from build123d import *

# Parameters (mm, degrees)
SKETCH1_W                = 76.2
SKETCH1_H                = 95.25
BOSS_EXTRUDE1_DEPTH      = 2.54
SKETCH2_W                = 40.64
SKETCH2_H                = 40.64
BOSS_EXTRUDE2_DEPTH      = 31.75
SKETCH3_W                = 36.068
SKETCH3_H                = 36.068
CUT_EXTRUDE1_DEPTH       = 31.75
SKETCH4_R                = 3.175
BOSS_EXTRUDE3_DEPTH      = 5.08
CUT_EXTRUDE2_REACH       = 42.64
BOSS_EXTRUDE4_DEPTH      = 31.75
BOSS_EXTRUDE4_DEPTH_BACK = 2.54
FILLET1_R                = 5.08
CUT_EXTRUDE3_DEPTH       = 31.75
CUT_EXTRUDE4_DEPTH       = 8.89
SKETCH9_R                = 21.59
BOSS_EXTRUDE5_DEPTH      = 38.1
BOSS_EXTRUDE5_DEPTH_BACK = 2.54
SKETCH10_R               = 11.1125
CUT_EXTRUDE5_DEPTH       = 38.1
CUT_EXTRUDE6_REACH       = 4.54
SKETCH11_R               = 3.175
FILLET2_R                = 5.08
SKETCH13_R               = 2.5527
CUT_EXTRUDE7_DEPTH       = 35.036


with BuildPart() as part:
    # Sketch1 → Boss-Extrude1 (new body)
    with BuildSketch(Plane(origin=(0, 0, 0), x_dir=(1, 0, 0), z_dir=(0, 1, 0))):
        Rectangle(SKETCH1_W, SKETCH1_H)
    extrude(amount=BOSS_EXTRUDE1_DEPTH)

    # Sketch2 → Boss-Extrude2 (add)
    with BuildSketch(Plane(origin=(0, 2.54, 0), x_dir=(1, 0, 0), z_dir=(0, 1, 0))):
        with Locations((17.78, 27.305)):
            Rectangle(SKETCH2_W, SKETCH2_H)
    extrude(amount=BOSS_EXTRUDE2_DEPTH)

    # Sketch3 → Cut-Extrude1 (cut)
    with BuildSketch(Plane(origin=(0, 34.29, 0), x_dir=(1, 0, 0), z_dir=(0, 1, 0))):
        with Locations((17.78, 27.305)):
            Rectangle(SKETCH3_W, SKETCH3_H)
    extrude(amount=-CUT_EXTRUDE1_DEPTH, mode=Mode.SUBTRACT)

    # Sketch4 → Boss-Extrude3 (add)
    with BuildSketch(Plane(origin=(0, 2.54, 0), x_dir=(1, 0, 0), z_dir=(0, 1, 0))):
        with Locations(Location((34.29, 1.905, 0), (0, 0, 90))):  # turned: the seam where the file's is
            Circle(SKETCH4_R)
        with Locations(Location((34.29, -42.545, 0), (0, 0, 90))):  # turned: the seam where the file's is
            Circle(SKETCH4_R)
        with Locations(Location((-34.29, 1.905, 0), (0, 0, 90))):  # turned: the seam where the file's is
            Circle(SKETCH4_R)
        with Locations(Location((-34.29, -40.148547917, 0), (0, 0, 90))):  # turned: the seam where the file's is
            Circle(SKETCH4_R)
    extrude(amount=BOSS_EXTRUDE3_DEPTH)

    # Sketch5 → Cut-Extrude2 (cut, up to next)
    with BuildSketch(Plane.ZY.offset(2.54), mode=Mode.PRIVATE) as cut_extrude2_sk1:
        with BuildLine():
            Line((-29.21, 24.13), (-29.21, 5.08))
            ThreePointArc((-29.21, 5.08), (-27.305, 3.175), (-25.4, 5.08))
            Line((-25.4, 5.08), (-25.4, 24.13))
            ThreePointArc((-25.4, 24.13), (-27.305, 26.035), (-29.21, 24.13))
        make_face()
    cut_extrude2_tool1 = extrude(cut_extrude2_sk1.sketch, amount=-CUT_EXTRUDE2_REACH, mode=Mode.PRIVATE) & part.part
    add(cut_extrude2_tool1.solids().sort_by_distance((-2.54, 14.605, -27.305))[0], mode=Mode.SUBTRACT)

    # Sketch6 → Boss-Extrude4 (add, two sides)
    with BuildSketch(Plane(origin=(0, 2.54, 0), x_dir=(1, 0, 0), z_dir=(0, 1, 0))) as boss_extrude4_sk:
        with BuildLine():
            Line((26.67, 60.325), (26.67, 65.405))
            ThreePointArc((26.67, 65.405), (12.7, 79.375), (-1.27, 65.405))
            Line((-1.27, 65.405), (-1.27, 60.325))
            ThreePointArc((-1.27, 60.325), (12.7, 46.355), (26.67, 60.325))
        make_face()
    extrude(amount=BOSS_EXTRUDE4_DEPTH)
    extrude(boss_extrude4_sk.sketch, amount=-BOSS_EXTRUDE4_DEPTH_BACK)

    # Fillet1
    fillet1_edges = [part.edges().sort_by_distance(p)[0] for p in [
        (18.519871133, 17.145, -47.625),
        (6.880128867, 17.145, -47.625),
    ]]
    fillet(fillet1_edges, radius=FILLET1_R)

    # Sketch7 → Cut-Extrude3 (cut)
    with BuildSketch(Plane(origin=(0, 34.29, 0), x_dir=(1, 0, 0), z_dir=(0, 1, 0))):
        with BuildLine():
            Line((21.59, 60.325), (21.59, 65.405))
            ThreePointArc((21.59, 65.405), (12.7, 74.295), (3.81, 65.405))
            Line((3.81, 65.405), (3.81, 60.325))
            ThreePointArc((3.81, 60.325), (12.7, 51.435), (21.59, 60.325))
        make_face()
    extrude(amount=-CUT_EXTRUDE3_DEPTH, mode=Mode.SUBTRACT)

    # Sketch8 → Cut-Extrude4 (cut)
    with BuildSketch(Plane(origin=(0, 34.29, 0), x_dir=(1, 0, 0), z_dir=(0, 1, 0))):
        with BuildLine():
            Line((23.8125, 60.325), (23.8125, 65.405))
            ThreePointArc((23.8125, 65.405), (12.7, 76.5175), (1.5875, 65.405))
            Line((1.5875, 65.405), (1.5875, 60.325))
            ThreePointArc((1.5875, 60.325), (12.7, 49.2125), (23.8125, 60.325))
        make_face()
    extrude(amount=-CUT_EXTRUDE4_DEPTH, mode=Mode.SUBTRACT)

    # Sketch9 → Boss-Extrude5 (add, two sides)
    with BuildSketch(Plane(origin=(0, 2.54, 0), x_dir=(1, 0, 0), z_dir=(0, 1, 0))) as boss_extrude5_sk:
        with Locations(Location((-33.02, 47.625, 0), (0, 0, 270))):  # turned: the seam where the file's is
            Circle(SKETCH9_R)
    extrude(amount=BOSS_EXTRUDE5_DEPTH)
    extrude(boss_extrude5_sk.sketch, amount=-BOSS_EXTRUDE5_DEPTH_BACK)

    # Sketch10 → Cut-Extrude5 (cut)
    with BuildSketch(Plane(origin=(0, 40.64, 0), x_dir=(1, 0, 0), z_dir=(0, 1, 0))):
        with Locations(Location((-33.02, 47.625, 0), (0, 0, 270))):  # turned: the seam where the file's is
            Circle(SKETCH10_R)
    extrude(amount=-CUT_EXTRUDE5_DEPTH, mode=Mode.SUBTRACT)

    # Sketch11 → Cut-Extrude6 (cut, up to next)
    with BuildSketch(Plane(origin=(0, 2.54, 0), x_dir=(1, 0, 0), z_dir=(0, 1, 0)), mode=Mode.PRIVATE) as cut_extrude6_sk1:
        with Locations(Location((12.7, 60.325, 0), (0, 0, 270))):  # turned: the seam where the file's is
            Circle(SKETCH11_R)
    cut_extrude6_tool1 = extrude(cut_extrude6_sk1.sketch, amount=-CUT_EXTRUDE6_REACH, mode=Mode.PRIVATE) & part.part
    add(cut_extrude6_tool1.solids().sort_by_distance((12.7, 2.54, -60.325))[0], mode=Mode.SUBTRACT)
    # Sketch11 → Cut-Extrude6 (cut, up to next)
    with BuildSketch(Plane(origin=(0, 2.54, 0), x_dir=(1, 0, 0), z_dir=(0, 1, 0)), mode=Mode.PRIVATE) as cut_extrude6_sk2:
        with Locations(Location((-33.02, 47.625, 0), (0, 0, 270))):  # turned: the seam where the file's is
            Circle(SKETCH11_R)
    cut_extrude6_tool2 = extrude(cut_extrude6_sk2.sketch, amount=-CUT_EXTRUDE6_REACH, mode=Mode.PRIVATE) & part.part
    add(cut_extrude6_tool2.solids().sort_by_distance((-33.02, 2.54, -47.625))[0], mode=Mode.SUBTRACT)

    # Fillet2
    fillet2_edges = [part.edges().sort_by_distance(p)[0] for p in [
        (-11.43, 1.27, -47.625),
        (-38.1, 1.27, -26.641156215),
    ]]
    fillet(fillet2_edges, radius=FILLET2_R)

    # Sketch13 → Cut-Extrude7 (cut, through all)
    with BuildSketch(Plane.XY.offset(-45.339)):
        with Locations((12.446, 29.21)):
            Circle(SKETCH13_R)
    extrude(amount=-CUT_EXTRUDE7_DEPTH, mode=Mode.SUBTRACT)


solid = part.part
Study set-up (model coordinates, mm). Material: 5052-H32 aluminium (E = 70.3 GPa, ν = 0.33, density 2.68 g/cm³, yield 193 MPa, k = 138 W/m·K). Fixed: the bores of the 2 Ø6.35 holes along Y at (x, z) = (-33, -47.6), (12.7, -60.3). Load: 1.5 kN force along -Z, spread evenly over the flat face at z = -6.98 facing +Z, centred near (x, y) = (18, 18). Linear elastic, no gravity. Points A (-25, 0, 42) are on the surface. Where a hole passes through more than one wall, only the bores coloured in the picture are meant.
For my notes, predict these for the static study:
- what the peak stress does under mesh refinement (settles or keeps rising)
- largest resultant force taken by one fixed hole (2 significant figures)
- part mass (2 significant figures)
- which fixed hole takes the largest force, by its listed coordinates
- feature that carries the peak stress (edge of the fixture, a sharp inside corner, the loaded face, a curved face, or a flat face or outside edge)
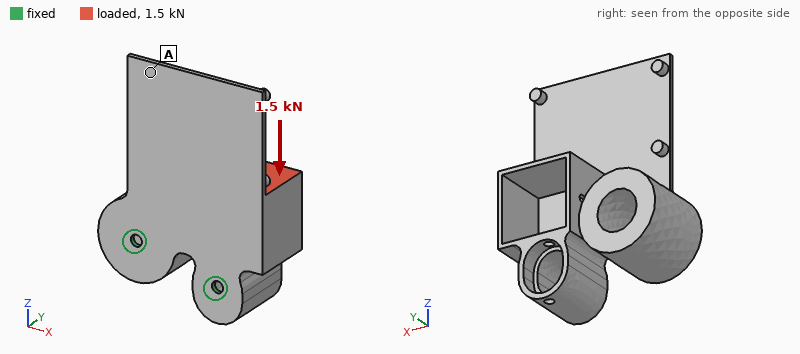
keeps rising
1.6 kN
240 g
(12.7, -60.3)
edge of the fixture
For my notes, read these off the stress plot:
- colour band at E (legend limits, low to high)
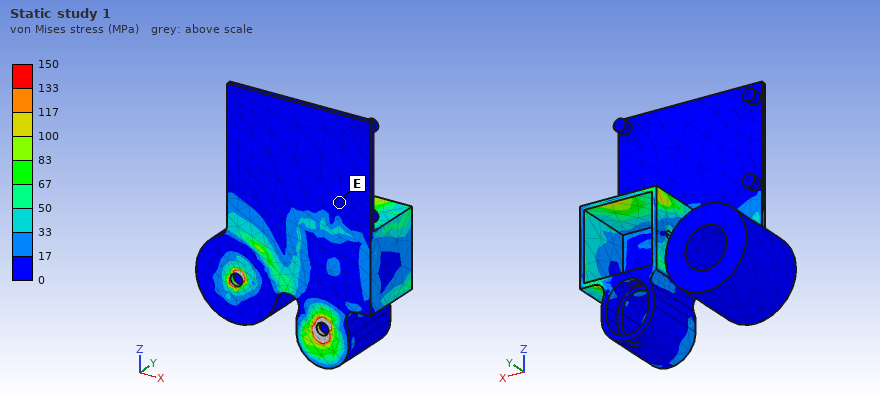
0 to 17 MPa
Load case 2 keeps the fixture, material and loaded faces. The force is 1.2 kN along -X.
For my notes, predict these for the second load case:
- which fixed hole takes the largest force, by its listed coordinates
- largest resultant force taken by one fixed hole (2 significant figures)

(-33, -47.6)
1.5 kN
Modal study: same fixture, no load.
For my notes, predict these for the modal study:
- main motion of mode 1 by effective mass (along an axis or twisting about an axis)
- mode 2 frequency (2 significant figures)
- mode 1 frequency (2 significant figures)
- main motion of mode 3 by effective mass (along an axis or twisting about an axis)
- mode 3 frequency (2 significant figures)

along Y
840 Hz
420 Hz
along Z
940 Hz
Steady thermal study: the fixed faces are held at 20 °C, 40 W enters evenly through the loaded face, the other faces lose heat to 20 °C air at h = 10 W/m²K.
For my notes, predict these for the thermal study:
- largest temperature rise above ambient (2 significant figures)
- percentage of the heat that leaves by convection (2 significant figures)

68 K
22 %
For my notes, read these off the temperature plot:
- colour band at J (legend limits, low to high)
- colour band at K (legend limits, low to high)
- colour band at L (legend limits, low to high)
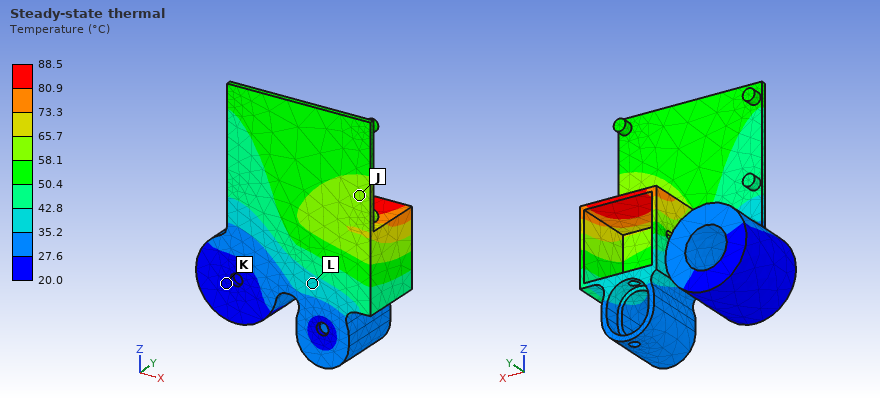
58.1 to 65.7 °C
20.0 to 27.6 °C
35.2 to 42.8 °C
